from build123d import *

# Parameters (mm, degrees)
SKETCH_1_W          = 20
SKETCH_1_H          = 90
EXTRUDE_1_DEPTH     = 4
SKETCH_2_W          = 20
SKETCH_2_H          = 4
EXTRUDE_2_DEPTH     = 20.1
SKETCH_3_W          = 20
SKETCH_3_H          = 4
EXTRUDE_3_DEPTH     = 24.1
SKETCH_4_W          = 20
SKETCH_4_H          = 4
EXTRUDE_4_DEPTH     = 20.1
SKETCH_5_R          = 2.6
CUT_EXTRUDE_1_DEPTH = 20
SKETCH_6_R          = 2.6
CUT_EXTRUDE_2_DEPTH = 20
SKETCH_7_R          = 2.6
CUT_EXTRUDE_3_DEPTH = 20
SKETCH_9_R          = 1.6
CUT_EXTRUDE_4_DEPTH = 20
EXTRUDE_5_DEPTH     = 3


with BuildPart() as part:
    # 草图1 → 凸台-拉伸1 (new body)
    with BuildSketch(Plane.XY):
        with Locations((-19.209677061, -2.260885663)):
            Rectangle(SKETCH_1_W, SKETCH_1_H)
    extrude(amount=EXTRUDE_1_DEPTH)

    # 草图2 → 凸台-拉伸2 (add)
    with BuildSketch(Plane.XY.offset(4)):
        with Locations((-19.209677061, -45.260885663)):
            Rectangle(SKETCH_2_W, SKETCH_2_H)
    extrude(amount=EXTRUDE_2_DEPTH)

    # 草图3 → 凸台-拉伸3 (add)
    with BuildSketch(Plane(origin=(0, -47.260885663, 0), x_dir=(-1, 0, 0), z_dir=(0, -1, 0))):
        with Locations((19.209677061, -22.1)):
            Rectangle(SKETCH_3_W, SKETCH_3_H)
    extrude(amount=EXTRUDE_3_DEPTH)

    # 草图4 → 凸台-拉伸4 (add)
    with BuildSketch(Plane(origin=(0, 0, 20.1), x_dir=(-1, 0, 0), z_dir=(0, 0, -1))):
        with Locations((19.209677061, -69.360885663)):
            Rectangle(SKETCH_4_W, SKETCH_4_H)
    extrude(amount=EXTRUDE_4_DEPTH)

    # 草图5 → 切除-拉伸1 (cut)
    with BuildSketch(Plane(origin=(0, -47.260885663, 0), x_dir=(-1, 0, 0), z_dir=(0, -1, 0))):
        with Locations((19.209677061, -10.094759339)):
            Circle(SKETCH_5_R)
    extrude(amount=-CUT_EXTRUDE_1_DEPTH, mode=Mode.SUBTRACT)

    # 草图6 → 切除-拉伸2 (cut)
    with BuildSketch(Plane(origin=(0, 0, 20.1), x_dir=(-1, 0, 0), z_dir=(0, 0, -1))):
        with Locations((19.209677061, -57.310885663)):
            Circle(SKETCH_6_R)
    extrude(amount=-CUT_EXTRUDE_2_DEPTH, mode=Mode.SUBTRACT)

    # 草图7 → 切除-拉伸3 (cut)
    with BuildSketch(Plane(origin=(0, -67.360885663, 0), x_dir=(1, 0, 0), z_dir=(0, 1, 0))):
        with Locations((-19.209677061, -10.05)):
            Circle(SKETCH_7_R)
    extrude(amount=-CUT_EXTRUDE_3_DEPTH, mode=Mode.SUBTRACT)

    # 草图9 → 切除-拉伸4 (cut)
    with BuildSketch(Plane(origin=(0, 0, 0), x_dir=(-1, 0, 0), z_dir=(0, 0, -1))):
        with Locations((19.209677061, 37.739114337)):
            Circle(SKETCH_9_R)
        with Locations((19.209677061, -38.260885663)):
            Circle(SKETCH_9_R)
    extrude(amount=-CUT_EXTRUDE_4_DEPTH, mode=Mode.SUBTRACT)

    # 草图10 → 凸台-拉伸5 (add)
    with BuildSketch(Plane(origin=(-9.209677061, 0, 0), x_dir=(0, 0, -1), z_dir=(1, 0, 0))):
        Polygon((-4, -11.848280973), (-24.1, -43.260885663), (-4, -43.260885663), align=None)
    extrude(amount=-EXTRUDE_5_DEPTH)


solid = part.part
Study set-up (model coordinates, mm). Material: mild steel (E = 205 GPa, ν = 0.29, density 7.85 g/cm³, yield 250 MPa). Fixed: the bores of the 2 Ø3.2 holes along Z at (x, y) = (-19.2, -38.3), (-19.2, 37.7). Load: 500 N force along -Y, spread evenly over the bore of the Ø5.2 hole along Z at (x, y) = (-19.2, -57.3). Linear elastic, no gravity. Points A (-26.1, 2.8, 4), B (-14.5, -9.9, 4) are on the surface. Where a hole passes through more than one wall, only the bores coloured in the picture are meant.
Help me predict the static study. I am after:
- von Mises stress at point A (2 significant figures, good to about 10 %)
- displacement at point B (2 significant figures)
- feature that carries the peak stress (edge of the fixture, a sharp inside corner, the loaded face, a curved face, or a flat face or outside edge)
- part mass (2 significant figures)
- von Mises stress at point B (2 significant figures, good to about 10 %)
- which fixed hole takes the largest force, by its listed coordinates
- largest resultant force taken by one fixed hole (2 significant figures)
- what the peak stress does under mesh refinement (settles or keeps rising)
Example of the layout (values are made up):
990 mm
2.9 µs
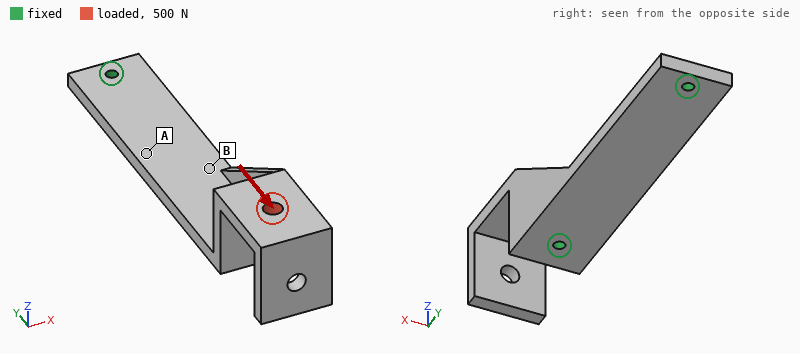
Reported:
15 MPa
24 µm
edge of the fixture
100 g
33 MPa
(-19.2, -38.3)
390 N
keeps rising
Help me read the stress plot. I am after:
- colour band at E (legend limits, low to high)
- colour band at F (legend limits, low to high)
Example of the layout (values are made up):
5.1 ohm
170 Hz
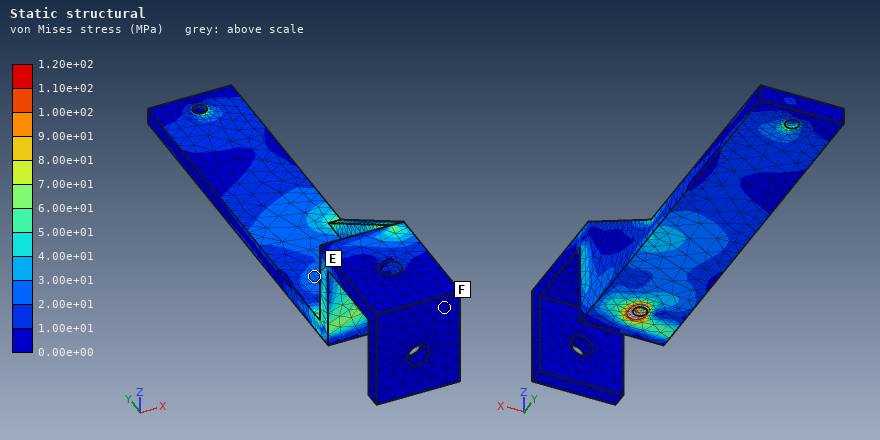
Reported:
2.00e+01 to 3.00e+01 MPa
0.00e+00 to 1.00e+01 MPa
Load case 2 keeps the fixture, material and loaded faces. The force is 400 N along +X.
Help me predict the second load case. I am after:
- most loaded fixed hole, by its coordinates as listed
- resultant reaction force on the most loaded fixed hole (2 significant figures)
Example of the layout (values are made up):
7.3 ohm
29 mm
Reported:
(-19.2, -38.3)
480 N
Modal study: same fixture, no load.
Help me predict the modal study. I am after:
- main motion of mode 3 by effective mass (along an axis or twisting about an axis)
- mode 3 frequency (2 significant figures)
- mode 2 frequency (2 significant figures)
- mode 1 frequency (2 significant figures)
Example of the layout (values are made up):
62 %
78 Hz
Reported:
along Y
2900 Hz
2000 Hz
1500 Hz
